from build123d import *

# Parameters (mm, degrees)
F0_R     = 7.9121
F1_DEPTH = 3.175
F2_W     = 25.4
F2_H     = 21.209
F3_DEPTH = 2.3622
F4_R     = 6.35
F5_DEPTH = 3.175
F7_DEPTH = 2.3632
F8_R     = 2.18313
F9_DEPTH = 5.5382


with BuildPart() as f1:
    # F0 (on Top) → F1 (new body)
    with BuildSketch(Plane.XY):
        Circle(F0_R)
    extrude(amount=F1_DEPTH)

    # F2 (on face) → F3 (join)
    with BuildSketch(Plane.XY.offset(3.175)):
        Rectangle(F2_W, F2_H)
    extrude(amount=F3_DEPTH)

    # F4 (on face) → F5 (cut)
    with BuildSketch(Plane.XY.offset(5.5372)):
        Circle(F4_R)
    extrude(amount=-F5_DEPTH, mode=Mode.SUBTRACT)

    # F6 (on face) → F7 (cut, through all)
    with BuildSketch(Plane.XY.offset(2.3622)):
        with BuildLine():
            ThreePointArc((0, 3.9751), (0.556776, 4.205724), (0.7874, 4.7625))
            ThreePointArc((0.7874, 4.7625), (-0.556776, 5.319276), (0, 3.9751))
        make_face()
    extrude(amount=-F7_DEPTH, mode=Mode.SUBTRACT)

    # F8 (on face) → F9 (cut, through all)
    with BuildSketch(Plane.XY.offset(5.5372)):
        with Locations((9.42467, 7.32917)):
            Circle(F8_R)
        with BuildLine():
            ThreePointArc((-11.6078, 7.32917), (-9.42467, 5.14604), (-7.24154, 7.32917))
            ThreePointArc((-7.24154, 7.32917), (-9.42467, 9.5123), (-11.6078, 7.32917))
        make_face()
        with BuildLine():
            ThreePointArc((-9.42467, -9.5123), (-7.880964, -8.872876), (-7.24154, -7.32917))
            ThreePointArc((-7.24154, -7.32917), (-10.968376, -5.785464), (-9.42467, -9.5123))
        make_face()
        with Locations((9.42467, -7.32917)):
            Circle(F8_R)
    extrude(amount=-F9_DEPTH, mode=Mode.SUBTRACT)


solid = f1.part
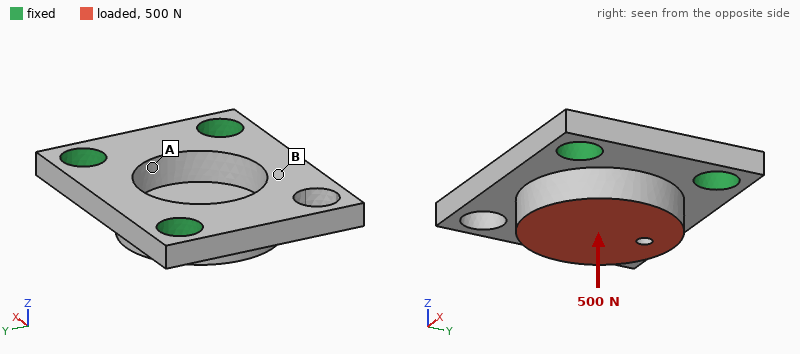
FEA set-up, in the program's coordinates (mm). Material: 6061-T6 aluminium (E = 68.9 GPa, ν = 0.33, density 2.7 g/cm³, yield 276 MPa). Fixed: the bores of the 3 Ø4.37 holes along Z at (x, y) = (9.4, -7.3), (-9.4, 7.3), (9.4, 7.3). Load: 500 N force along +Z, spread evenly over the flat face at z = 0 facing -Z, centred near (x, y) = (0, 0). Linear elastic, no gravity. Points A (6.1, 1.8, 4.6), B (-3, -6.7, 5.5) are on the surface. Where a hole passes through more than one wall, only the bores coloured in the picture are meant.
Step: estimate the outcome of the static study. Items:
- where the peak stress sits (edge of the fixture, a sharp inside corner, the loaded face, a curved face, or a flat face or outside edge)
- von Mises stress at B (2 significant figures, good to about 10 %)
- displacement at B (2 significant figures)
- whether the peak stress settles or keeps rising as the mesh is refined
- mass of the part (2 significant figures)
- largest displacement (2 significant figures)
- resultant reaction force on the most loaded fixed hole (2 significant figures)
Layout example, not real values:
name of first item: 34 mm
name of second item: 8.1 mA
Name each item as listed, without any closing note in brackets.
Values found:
where the peak stress sits: edge of the fixture
von Mises stress at B: 15 MPa
displacement at B: 11 µm
whether the peak stress settles or keeps rising as the mesh is refined: keeps rising
mass of the part: 3.6 g
largest displacement: 19 µm
resultant reaction force on the most loaded fixed hole: 290 N
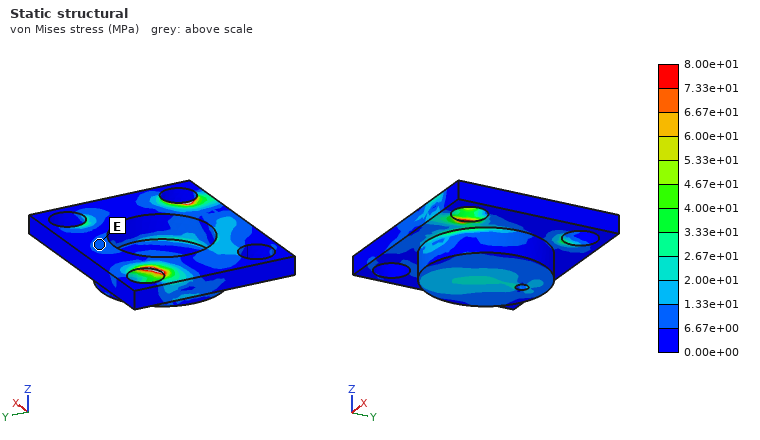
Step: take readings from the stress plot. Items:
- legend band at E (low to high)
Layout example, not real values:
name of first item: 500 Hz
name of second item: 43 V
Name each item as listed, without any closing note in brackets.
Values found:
legend band at E: 6.67e+00 to 1.33e+01 MPa
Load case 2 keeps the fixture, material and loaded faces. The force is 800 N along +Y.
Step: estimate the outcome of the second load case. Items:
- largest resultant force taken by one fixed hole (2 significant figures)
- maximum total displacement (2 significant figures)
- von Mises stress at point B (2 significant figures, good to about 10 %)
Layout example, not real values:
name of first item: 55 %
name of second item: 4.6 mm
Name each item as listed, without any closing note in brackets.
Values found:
largest resultant force taken by one fixed hole: 390 N
maximum total displacement: 23 µm
von Mises stress at point B: 12 MPa
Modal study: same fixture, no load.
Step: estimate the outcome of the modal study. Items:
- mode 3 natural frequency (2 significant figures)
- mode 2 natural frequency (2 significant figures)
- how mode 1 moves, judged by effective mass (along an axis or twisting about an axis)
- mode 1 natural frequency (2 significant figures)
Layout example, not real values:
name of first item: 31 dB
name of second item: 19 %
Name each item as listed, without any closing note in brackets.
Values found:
mode 3 natural frequency: 44 kHz
mode 2 natural frequency: 35 kHz
how mode 1 moves, judged by effective mass: along Z
mode 1 natural frequency: 16 kHz
